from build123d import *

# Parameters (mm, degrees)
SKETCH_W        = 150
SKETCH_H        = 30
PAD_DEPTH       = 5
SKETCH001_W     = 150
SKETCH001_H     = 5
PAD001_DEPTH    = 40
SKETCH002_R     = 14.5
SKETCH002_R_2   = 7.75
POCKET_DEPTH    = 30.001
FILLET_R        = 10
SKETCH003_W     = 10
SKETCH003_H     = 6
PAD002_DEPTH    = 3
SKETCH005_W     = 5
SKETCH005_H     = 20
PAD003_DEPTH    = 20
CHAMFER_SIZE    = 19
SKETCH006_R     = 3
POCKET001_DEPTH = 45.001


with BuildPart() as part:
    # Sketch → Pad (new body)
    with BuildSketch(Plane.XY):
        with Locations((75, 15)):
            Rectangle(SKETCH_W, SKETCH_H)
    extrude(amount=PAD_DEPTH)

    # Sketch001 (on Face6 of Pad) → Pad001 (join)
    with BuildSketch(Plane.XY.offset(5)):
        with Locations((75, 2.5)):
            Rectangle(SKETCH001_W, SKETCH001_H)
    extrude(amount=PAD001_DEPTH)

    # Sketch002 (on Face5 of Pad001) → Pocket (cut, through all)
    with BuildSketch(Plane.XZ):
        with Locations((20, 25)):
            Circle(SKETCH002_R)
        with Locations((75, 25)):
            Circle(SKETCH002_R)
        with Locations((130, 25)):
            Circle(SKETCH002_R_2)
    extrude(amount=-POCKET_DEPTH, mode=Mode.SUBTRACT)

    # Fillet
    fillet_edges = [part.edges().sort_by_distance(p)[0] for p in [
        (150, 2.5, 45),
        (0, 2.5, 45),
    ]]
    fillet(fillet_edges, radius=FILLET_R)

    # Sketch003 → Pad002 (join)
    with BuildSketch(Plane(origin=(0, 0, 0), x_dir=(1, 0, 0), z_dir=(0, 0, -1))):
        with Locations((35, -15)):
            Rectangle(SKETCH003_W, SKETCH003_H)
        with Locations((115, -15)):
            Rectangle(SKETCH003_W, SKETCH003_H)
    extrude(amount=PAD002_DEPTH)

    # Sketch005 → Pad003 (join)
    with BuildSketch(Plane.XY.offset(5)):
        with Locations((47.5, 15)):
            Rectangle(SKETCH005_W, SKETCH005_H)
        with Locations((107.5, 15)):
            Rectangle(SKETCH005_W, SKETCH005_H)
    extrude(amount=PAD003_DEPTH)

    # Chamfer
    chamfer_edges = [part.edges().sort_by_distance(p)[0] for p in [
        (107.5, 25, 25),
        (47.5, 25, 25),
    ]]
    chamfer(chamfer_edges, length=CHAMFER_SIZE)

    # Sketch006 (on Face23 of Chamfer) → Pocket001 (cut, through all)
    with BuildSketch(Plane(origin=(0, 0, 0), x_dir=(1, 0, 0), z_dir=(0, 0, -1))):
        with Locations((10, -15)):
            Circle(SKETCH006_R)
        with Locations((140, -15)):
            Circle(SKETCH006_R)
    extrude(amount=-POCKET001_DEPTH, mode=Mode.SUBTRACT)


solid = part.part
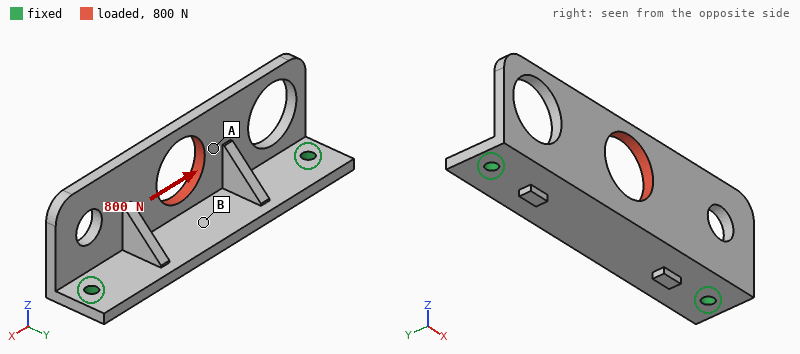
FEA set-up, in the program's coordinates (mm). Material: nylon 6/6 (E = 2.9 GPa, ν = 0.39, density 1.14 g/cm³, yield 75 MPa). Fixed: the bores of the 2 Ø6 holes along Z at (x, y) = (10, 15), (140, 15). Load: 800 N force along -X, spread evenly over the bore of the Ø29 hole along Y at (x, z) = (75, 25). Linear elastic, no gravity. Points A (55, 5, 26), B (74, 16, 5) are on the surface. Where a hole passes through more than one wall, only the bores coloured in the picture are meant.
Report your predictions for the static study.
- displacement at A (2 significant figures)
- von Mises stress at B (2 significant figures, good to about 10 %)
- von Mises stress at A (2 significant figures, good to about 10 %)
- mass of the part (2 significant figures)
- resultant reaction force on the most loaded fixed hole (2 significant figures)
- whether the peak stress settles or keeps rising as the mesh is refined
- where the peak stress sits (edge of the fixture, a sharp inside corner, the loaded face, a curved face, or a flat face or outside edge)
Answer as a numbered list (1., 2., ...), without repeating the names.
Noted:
1. 0.14 mm
2. 1.3 MPa
3. 3.7 MPa
4. 54 g
5. 430 N
6. keeps rising
7. edge of the fixture
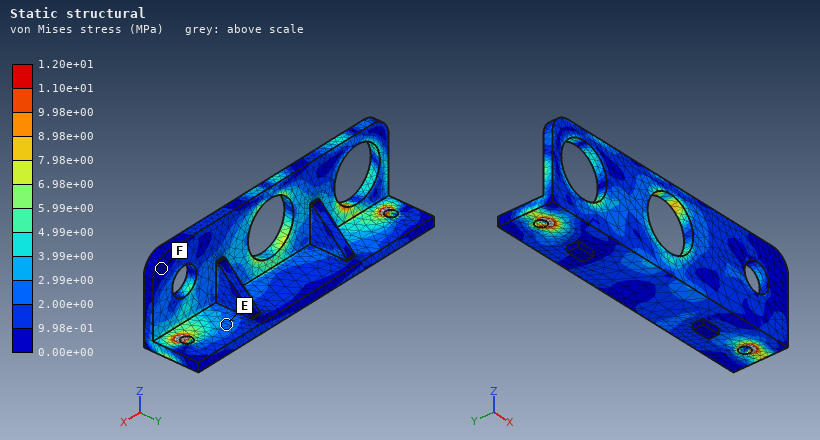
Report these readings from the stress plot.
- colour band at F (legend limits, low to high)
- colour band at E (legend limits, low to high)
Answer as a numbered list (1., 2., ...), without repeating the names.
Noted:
1. 0.00e+00 to 9.98e-01 MPa
2. 2.00e+00 to 2.99e+00 MPa
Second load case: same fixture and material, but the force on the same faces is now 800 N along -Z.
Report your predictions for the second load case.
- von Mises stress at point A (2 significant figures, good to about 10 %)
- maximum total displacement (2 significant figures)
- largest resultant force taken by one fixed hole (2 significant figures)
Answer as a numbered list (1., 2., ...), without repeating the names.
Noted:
1. 5.6 MPa
2. 1.7 mm
3. 490 N
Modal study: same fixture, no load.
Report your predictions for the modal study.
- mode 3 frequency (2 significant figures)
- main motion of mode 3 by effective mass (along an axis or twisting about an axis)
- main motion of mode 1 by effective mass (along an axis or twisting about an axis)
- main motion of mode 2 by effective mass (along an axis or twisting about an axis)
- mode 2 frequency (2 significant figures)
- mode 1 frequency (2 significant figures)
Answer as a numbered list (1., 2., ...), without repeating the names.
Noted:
1. 940 Hz
2. along Z
3. along Y
4. twisting about Z
5. 690 Hz
6. 420 Hz
